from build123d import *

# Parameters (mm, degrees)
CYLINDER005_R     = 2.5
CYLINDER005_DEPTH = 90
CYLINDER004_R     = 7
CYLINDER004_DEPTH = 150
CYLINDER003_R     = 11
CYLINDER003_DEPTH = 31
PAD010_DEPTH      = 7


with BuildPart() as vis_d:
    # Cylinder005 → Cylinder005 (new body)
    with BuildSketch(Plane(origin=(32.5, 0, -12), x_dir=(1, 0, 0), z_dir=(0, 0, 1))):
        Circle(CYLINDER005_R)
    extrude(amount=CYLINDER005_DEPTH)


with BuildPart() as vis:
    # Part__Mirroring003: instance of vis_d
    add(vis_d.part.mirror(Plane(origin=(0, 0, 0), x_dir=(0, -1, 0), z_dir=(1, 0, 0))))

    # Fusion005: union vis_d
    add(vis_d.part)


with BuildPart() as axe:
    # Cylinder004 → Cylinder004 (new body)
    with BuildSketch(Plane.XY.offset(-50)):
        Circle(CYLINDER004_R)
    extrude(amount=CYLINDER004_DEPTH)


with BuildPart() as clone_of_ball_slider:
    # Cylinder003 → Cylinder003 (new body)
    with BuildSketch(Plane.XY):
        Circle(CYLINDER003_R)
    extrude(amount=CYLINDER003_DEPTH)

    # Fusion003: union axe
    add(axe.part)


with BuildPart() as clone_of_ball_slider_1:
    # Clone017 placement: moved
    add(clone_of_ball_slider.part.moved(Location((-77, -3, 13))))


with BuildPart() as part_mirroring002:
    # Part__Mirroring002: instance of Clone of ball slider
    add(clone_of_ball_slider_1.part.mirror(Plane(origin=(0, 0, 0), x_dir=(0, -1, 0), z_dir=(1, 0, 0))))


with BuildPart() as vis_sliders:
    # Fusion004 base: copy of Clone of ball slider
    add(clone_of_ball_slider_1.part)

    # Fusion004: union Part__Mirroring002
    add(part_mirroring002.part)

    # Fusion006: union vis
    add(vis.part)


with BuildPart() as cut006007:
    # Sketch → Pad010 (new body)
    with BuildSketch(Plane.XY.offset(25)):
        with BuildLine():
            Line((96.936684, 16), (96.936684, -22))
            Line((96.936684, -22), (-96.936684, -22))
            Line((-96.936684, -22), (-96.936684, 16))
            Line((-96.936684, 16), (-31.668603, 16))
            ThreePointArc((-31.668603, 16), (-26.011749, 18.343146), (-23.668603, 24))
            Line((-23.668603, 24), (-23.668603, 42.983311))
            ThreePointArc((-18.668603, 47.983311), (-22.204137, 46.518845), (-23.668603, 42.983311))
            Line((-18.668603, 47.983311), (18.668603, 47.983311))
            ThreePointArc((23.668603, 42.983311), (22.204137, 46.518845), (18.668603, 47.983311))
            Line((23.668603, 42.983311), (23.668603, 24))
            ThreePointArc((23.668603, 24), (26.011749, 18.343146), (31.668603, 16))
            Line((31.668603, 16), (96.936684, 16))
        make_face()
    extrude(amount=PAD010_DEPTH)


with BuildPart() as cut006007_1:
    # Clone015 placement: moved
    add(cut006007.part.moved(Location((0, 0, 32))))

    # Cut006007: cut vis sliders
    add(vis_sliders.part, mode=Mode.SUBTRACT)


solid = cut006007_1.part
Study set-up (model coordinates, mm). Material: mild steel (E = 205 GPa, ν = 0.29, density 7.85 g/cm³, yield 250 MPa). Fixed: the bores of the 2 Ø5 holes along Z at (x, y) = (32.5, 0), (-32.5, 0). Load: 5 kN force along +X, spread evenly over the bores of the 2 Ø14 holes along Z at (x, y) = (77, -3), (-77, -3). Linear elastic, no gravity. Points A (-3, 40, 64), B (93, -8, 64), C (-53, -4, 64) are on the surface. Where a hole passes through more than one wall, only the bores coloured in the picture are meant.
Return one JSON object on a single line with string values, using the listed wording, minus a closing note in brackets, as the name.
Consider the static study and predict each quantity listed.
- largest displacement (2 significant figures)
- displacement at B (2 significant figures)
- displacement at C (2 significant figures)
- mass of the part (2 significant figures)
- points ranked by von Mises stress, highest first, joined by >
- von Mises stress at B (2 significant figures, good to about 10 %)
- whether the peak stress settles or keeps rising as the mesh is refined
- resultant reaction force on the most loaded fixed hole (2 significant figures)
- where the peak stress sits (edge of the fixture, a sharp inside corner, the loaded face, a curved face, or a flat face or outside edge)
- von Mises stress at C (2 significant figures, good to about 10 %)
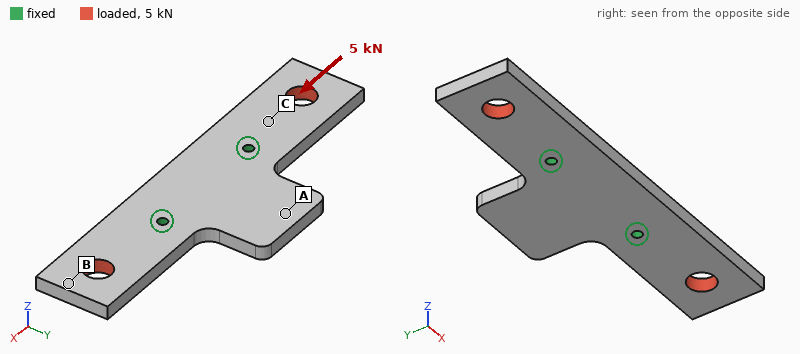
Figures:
{"largest displacement": "4.0 µm", "displacement at B": "3.8 µm", "displacement at C": "1.6 µm", "mass of the part": "470 g", "points ranked by von Mises stress, highest first, joined by >": "C > B > A", "von Mises stress at B": "5.9 MPa", "whether the peak stress settles or keeps rising as the mesh is refined": "keeps rising", "resultant reaction force on the most loaded fixed hole": "2.5 kN", "where the peak stress sits": "edge of the fixture", "von Mises stress at C": "11 MPa"}
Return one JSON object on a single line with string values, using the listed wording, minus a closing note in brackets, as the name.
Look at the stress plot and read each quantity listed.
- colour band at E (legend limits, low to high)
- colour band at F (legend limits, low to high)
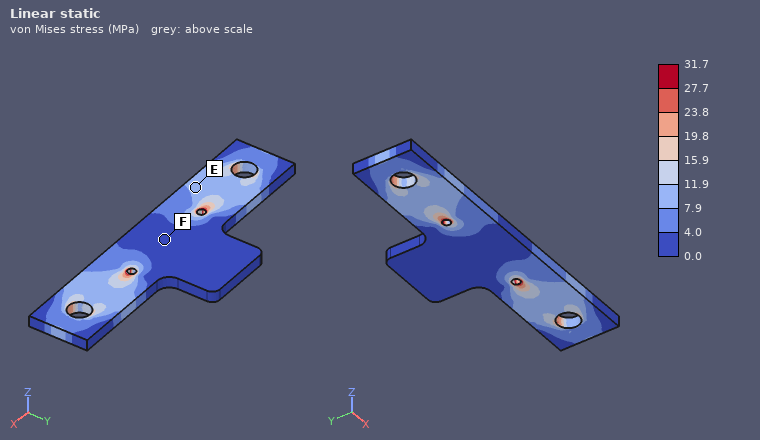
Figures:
{"colour band at E": "7.9 to 11.9 MPa", "colour band at F": "0.0 to 4.0 MPa"}
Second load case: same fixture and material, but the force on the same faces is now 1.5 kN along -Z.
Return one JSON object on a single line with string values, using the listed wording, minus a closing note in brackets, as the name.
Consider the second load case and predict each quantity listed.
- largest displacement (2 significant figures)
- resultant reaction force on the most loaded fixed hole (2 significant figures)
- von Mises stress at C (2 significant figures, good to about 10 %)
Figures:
{"largest displacement": "0.19 mm", "resultant reaction force on the most loaded fixed hole": "750 N", "von Mises stress at C": "53 MPa"}
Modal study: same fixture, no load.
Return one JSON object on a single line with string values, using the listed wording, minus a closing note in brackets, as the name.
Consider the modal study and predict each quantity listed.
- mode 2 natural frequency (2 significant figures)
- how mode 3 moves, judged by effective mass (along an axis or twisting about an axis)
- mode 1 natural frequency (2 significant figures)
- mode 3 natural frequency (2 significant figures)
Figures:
{"mode 2 natural frequency": "1400 Hz", "how mode 3 moves, judged by effective mass": "along Z", "mode 1 natural frequency": "1300 Hz", "mode 3 natural frequency": "2200 Hz"}
